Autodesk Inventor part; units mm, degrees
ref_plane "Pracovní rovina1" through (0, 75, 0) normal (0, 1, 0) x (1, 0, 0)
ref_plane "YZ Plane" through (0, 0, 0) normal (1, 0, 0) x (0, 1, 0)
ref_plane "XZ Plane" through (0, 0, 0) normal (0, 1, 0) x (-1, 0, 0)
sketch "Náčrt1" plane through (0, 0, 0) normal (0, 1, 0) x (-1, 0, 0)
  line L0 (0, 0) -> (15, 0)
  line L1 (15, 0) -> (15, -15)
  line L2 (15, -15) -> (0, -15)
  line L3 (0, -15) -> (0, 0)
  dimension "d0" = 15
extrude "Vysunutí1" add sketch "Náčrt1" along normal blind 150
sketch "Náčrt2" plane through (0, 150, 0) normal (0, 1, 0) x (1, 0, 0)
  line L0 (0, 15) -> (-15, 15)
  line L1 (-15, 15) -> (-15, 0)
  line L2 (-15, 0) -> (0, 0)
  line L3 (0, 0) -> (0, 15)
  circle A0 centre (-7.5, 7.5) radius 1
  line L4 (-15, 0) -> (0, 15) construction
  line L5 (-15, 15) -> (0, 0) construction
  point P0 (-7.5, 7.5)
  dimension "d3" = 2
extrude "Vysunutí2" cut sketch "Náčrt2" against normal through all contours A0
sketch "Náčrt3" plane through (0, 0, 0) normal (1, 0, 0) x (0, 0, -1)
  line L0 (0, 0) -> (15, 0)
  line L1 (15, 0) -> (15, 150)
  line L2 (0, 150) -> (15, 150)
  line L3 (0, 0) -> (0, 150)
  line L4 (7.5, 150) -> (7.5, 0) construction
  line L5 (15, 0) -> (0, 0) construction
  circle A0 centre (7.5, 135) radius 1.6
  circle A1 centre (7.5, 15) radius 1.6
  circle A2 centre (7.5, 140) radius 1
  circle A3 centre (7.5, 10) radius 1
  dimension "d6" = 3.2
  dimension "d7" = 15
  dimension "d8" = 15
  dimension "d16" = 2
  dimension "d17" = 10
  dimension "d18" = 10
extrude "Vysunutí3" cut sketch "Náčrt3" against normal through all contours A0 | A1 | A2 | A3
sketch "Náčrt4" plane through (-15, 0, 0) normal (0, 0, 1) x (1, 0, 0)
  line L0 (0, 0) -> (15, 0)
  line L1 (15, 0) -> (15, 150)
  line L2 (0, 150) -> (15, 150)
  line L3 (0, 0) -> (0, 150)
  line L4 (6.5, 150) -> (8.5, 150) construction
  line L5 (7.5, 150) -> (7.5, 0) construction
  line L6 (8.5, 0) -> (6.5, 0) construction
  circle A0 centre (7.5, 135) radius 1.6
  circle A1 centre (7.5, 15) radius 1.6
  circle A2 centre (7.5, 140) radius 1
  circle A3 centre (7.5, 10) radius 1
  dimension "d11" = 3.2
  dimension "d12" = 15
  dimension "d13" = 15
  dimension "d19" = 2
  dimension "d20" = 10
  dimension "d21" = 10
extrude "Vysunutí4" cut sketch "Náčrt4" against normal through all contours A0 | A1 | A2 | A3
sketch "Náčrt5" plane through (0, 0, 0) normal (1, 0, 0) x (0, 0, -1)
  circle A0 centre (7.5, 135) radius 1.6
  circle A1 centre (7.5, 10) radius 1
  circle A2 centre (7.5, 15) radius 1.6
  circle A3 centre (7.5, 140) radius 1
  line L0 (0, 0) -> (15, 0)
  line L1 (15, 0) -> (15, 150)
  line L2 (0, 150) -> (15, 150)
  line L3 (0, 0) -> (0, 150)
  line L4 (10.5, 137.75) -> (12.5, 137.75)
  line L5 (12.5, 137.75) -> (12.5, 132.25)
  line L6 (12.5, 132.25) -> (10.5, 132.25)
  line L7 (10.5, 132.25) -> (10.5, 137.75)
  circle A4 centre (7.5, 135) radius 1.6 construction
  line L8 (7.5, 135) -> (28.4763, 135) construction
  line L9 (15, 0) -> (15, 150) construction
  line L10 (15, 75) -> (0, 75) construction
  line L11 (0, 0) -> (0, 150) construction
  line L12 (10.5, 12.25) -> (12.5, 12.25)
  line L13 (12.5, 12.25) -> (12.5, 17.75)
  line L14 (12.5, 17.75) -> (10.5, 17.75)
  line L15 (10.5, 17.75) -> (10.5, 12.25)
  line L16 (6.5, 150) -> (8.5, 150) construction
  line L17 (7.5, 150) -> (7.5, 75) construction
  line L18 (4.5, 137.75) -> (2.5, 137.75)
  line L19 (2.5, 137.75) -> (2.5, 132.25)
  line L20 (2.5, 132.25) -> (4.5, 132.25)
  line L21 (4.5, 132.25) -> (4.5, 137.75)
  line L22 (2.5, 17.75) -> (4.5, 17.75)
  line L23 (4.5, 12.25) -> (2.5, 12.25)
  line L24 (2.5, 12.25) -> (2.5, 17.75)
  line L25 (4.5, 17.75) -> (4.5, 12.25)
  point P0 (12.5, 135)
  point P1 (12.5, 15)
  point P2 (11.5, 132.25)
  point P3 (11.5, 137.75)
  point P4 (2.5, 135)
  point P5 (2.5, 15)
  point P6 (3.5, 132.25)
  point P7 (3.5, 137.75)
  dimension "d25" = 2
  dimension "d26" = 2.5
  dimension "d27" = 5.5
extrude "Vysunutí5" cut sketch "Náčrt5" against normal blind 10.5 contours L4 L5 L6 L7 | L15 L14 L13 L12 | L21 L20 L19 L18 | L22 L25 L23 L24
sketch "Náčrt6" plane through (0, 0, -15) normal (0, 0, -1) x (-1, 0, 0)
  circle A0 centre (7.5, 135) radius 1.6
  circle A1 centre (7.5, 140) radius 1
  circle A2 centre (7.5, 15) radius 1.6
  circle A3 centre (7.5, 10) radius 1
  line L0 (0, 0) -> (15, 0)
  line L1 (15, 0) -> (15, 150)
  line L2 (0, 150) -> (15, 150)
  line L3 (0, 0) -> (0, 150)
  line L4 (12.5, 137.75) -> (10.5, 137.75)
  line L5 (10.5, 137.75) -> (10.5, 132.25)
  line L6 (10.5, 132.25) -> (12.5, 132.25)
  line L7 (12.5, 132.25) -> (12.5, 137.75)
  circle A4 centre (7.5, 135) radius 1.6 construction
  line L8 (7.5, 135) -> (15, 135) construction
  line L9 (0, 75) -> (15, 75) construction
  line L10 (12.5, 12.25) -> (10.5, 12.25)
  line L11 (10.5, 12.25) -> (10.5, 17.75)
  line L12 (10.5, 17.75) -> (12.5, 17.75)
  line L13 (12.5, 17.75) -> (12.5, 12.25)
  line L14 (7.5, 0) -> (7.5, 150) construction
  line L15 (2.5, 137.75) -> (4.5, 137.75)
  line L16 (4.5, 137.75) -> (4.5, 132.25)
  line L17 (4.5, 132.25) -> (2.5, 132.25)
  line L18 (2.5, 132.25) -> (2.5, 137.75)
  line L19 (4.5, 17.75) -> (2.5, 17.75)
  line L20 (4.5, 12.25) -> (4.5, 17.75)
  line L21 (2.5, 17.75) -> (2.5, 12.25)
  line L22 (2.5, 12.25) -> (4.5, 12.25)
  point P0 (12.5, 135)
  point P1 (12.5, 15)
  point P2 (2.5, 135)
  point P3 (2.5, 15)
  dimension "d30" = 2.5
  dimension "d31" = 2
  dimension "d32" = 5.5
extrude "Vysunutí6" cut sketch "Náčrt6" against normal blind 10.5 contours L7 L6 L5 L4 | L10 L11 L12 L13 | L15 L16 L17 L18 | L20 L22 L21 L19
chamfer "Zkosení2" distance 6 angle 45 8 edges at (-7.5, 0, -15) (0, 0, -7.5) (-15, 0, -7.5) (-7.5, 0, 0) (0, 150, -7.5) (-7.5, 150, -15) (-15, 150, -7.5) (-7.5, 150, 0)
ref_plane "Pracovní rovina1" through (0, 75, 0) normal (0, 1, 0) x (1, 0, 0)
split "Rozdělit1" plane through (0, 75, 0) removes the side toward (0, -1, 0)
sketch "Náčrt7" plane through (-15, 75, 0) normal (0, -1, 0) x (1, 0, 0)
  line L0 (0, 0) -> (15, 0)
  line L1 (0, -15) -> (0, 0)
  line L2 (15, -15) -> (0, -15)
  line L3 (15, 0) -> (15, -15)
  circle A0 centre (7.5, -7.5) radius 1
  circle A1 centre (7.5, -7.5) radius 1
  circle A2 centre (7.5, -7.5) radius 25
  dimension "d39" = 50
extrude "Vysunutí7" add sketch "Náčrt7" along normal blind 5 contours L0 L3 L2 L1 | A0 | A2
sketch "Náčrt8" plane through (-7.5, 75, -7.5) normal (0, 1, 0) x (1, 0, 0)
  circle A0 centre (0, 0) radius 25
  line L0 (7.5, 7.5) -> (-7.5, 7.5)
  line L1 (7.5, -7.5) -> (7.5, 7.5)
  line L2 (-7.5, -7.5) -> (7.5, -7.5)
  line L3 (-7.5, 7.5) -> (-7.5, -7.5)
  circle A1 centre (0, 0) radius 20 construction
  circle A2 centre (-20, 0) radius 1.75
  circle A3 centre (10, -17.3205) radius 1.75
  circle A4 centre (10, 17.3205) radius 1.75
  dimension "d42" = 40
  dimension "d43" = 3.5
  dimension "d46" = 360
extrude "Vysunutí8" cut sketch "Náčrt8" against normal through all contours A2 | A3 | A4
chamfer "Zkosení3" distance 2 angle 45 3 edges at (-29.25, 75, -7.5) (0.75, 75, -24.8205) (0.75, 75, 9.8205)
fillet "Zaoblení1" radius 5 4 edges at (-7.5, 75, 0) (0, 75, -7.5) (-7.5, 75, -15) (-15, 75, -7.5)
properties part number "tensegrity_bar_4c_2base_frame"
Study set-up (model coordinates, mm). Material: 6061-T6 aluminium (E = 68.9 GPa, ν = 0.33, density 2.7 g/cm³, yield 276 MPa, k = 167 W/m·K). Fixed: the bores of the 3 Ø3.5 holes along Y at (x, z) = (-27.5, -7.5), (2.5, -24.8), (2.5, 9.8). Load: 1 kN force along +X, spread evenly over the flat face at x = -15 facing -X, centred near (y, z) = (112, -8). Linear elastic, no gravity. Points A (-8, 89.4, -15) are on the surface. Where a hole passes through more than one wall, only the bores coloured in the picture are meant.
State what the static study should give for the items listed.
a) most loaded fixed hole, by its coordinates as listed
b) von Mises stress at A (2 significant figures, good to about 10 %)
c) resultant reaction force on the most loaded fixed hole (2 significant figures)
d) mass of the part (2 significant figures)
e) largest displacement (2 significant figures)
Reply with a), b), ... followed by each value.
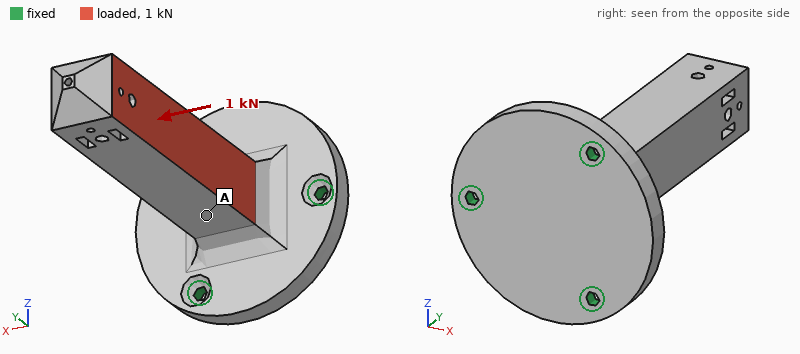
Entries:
a) (-27.5, -7.5)
b) 12 MPa
c) 1.6 kN
d) 68 g
e) 0.30 mm
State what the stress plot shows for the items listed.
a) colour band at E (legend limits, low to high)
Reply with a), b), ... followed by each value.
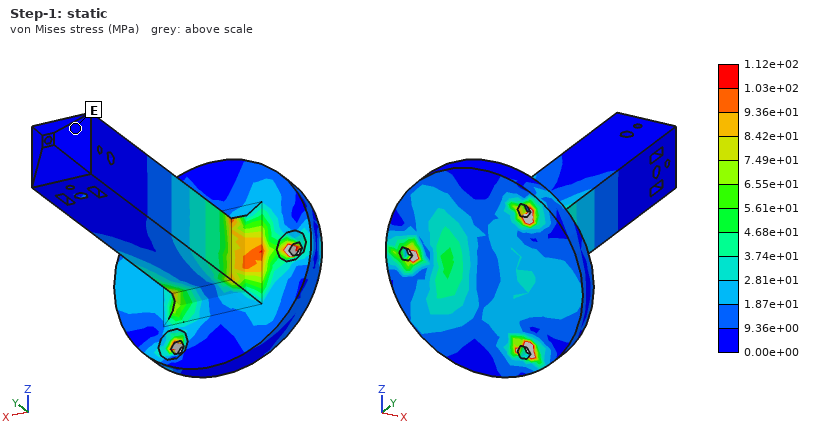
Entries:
a) 0.00e+00 to 9.36e+00 MPa
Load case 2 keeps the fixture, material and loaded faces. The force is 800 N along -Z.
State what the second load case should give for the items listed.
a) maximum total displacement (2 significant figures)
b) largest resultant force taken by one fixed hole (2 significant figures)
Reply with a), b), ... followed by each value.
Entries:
a) 0.24 mm
b) 1.1 kN
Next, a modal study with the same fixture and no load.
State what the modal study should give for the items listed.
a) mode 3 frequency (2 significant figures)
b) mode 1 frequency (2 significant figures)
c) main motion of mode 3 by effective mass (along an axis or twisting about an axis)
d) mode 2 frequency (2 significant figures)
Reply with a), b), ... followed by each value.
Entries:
a) 7900 Hz
b) 1900 Hz
c) along Y
d) 1900 Hz
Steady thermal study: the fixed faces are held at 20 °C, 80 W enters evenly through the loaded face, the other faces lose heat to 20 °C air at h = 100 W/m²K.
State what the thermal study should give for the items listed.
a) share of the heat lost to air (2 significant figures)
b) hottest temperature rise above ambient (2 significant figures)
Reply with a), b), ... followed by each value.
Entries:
a) 35 %
b) 68 K
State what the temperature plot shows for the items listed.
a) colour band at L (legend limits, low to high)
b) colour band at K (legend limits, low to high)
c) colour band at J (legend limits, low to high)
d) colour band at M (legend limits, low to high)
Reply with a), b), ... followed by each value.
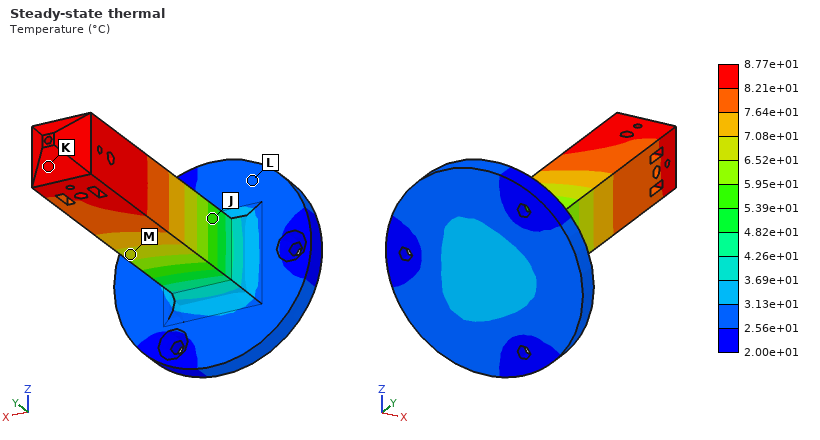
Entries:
a) 2.56e+01 to 3.13e+01 °C
b) 8.21e+01 to 8.77e+01 °C
c) 5.39e+01 to 5.95e+01 °C
d) 6.52e+01 to 7.08e+01 °C
